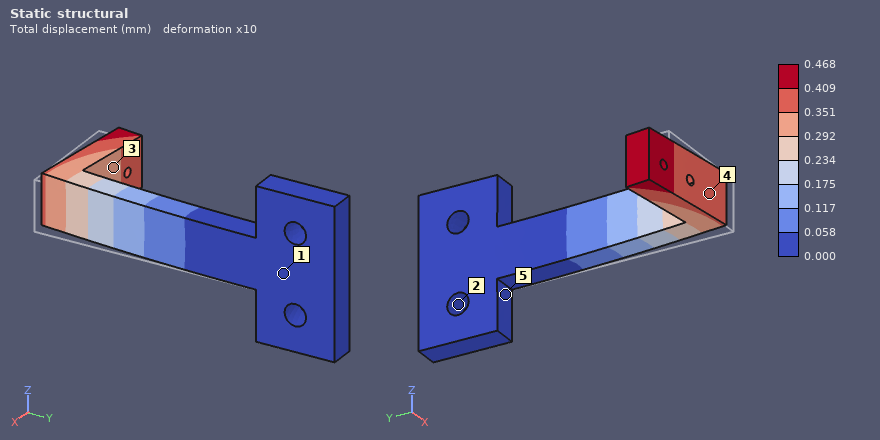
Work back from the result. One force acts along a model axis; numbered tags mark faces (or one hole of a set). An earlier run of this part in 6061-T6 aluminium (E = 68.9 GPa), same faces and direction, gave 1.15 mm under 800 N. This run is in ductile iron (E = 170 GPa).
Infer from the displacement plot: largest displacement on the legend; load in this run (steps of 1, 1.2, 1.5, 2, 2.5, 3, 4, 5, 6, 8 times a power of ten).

0.468 mm
800 N
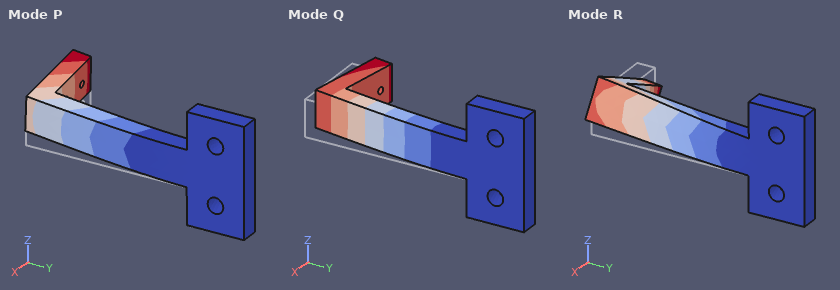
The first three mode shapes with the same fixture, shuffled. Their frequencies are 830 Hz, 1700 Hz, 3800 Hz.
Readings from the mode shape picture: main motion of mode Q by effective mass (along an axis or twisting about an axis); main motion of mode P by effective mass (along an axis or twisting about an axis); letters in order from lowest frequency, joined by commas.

along X
along Z
Q, P, R
